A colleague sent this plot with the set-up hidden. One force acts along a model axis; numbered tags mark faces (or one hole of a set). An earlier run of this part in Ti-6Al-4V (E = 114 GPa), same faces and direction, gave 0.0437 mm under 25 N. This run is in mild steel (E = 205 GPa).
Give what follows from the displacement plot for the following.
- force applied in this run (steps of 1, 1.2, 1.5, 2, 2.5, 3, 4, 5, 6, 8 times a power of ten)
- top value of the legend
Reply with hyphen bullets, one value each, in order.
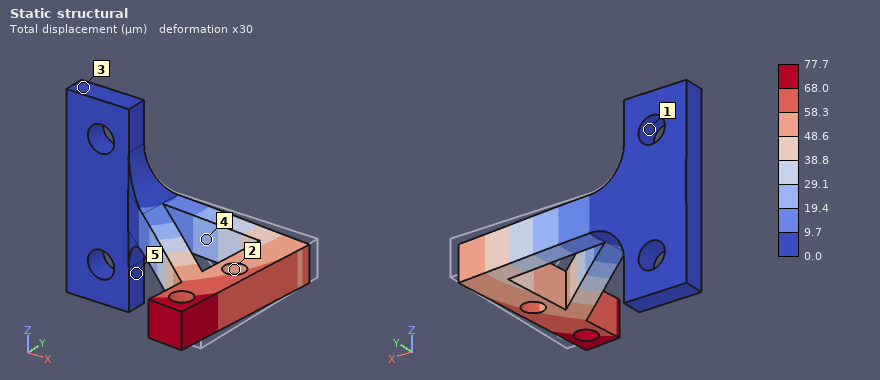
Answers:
- 80 N
- 77.7 µm
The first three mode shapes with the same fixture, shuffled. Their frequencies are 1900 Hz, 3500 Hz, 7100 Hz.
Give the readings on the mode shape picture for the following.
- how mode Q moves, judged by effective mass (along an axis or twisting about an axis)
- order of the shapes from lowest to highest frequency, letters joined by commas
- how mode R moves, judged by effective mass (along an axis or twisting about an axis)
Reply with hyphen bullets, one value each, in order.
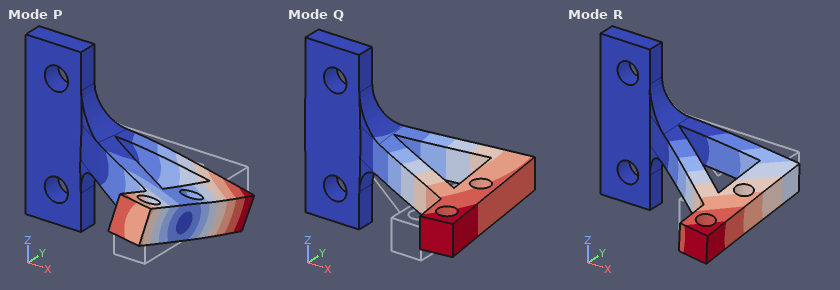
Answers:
- along Y
- Q, R, P
- along Z
